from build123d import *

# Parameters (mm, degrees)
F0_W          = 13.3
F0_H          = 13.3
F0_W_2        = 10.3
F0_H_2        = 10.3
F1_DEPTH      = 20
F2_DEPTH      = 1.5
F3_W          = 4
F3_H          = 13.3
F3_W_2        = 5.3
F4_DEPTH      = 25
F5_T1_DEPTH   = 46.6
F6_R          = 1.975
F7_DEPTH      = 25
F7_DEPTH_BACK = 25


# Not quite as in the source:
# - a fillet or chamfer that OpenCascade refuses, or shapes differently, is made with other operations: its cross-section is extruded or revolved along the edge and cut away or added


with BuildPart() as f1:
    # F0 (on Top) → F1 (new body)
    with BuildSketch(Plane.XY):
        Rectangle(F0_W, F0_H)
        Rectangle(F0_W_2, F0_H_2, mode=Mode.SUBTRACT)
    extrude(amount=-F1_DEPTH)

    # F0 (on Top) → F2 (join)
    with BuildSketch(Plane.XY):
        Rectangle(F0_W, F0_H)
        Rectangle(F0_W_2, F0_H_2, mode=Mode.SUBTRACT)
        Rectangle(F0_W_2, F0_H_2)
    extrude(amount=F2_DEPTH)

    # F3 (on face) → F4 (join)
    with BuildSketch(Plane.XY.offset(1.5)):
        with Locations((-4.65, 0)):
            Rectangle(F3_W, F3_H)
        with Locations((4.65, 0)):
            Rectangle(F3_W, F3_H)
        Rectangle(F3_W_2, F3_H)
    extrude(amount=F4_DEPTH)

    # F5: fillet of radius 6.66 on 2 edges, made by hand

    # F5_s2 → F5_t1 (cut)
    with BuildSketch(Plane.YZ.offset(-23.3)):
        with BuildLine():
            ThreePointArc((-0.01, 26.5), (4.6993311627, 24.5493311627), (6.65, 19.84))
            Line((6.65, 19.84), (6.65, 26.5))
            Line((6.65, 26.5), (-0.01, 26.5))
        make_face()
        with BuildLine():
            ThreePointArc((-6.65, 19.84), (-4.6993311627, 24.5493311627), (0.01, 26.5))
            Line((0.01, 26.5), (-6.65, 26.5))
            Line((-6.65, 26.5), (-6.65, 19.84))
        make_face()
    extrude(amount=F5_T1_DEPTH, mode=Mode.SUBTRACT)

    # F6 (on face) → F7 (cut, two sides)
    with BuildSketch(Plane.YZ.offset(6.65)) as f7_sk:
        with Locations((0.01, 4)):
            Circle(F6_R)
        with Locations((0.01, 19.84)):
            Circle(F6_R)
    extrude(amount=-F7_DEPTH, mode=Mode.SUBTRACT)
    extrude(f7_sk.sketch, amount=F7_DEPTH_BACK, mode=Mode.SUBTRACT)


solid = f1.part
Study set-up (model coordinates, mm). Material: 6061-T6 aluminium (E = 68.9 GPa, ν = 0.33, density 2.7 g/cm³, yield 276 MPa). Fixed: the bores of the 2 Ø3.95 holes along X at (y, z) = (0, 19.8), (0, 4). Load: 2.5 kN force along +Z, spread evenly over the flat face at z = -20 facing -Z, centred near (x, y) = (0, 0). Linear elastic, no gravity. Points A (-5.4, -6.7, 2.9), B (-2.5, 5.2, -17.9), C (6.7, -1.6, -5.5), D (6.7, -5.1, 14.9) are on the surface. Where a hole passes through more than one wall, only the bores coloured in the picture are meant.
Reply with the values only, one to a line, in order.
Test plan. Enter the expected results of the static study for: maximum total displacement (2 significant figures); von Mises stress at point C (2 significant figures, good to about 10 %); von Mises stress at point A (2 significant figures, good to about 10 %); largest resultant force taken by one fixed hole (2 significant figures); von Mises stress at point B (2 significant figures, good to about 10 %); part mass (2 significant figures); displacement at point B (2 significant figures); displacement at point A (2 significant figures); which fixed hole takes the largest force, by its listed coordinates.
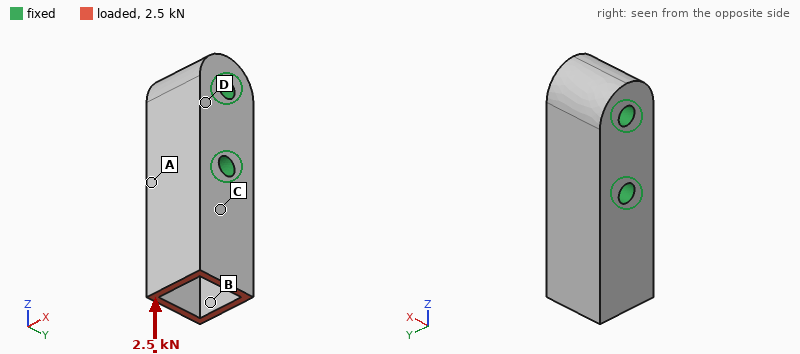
13 µm
40 MPa
22 MPa
2.1 kN
35 MPa
15 g
11 µm
2.0 µm
(0, 4)
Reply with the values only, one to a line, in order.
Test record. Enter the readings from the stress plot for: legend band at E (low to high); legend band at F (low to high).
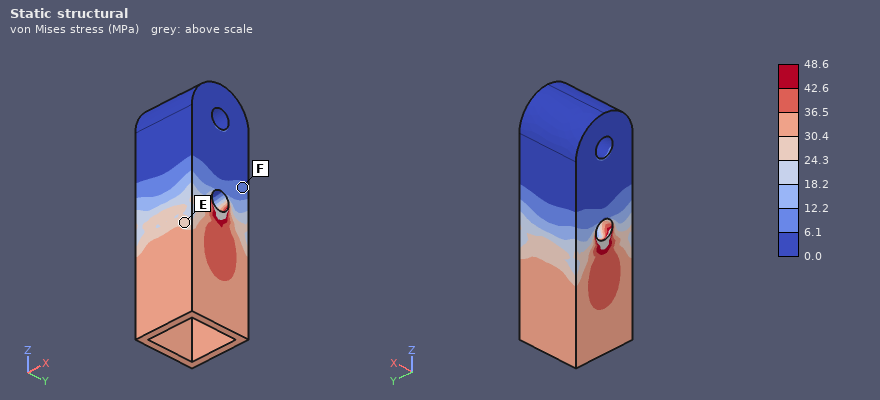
24.3 to 30.4 MPa
6.1 to 12.2 MPa
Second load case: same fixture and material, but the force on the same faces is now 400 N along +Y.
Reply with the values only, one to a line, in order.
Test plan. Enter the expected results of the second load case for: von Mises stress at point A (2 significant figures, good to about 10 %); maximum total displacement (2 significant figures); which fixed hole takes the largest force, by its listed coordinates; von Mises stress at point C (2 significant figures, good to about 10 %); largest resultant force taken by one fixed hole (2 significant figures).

29 MPa
45 µm
(0, 4)
23 MPa
730 N
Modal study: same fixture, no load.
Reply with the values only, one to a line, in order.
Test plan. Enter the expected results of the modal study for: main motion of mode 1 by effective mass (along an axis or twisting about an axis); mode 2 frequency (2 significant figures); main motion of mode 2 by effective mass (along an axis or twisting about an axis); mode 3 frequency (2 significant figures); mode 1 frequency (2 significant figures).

along Y
16 kHz
along X
20 kHz
15 kHz
